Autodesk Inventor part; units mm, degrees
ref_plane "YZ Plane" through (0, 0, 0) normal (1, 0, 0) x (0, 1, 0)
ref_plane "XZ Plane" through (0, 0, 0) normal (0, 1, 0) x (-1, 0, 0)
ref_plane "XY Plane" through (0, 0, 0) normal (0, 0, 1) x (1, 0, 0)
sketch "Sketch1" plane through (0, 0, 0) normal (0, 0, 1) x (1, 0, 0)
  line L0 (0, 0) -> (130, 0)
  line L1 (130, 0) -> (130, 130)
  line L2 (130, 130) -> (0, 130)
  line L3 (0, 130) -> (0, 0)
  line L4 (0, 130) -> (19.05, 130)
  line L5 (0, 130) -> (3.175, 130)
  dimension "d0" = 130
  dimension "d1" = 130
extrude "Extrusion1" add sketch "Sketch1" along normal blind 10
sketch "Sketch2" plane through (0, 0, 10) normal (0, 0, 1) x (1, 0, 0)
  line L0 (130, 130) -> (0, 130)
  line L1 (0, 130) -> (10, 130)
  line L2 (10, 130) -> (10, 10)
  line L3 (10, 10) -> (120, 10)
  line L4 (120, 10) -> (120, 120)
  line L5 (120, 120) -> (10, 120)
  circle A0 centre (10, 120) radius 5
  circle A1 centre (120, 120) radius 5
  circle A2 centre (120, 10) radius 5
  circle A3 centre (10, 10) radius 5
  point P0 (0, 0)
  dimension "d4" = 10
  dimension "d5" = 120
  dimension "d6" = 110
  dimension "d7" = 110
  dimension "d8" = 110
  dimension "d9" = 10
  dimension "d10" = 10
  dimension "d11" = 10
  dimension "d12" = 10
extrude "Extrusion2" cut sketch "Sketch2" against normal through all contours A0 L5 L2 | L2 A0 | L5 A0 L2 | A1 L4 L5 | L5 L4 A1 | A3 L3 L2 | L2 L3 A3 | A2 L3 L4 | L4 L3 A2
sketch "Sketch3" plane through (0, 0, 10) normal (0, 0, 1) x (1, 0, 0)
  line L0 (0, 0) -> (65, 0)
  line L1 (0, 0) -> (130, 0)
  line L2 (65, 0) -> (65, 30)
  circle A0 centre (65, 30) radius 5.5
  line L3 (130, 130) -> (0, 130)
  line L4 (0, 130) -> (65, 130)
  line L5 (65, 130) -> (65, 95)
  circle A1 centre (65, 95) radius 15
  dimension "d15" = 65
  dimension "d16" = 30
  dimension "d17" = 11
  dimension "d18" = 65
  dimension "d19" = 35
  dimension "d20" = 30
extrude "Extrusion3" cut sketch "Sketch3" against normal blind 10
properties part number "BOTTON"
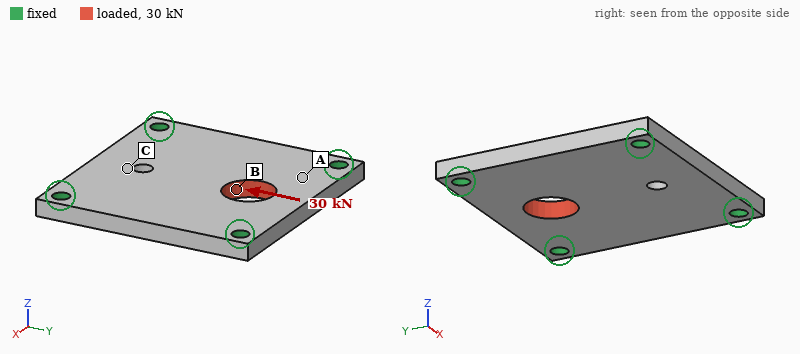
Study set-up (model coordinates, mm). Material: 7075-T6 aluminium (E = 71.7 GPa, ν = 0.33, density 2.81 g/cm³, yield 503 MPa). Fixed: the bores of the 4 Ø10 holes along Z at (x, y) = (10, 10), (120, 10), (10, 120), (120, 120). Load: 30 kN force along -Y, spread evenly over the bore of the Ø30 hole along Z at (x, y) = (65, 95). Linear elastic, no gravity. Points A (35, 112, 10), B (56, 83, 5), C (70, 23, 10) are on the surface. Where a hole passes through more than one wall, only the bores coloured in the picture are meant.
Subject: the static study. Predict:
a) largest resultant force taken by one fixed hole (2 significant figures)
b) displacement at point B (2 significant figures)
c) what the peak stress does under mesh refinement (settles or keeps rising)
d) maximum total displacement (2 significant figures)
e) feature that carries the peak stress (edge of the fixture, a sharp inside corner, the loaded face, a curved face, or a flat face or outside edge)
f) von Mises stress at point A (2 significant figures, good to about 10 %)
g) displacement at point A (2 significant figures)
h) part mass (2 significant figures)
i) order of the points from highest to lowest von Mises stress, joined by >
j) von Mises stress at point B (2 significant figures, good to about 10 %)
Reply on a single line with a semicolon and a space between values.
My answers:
8.8 kN; 31 µm; keeps rising; 55 µm; edge of the fixture; 26 MPa; 24 µm; 440 g; B > A > C; 42 MPa
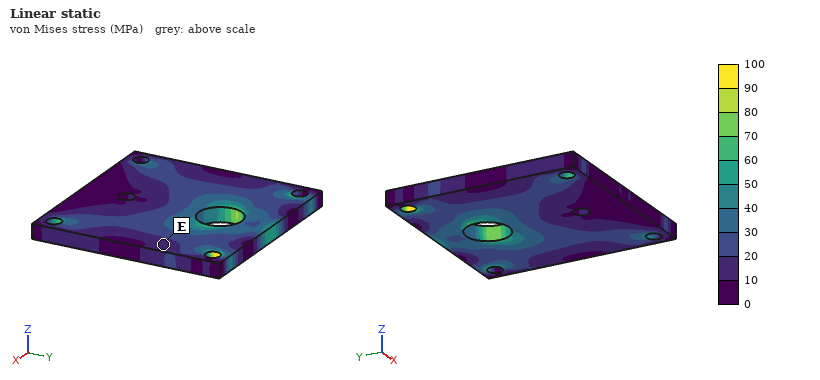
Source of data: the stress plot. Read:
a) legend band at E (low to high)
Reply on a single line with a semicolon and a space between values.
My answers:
10 to 20 MPa
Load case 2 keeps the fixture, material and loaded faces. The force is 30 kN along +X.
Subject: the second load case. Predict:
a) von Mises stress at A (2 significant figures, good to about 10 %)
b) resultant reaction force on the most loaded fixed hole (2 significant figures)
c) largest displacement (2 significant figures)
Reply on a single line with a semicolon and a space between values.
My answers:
33 MPa; 11 kN; 32 µm
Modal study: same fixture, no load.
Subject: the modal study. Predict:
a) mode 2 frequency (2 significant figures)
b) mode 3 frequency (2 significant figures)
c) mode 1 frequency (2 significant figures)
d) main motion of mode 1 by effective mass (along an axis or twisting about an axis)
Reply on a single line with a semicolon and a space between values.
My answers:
4700 Hz; 4800 Hz; 2800 Hz; along Z
